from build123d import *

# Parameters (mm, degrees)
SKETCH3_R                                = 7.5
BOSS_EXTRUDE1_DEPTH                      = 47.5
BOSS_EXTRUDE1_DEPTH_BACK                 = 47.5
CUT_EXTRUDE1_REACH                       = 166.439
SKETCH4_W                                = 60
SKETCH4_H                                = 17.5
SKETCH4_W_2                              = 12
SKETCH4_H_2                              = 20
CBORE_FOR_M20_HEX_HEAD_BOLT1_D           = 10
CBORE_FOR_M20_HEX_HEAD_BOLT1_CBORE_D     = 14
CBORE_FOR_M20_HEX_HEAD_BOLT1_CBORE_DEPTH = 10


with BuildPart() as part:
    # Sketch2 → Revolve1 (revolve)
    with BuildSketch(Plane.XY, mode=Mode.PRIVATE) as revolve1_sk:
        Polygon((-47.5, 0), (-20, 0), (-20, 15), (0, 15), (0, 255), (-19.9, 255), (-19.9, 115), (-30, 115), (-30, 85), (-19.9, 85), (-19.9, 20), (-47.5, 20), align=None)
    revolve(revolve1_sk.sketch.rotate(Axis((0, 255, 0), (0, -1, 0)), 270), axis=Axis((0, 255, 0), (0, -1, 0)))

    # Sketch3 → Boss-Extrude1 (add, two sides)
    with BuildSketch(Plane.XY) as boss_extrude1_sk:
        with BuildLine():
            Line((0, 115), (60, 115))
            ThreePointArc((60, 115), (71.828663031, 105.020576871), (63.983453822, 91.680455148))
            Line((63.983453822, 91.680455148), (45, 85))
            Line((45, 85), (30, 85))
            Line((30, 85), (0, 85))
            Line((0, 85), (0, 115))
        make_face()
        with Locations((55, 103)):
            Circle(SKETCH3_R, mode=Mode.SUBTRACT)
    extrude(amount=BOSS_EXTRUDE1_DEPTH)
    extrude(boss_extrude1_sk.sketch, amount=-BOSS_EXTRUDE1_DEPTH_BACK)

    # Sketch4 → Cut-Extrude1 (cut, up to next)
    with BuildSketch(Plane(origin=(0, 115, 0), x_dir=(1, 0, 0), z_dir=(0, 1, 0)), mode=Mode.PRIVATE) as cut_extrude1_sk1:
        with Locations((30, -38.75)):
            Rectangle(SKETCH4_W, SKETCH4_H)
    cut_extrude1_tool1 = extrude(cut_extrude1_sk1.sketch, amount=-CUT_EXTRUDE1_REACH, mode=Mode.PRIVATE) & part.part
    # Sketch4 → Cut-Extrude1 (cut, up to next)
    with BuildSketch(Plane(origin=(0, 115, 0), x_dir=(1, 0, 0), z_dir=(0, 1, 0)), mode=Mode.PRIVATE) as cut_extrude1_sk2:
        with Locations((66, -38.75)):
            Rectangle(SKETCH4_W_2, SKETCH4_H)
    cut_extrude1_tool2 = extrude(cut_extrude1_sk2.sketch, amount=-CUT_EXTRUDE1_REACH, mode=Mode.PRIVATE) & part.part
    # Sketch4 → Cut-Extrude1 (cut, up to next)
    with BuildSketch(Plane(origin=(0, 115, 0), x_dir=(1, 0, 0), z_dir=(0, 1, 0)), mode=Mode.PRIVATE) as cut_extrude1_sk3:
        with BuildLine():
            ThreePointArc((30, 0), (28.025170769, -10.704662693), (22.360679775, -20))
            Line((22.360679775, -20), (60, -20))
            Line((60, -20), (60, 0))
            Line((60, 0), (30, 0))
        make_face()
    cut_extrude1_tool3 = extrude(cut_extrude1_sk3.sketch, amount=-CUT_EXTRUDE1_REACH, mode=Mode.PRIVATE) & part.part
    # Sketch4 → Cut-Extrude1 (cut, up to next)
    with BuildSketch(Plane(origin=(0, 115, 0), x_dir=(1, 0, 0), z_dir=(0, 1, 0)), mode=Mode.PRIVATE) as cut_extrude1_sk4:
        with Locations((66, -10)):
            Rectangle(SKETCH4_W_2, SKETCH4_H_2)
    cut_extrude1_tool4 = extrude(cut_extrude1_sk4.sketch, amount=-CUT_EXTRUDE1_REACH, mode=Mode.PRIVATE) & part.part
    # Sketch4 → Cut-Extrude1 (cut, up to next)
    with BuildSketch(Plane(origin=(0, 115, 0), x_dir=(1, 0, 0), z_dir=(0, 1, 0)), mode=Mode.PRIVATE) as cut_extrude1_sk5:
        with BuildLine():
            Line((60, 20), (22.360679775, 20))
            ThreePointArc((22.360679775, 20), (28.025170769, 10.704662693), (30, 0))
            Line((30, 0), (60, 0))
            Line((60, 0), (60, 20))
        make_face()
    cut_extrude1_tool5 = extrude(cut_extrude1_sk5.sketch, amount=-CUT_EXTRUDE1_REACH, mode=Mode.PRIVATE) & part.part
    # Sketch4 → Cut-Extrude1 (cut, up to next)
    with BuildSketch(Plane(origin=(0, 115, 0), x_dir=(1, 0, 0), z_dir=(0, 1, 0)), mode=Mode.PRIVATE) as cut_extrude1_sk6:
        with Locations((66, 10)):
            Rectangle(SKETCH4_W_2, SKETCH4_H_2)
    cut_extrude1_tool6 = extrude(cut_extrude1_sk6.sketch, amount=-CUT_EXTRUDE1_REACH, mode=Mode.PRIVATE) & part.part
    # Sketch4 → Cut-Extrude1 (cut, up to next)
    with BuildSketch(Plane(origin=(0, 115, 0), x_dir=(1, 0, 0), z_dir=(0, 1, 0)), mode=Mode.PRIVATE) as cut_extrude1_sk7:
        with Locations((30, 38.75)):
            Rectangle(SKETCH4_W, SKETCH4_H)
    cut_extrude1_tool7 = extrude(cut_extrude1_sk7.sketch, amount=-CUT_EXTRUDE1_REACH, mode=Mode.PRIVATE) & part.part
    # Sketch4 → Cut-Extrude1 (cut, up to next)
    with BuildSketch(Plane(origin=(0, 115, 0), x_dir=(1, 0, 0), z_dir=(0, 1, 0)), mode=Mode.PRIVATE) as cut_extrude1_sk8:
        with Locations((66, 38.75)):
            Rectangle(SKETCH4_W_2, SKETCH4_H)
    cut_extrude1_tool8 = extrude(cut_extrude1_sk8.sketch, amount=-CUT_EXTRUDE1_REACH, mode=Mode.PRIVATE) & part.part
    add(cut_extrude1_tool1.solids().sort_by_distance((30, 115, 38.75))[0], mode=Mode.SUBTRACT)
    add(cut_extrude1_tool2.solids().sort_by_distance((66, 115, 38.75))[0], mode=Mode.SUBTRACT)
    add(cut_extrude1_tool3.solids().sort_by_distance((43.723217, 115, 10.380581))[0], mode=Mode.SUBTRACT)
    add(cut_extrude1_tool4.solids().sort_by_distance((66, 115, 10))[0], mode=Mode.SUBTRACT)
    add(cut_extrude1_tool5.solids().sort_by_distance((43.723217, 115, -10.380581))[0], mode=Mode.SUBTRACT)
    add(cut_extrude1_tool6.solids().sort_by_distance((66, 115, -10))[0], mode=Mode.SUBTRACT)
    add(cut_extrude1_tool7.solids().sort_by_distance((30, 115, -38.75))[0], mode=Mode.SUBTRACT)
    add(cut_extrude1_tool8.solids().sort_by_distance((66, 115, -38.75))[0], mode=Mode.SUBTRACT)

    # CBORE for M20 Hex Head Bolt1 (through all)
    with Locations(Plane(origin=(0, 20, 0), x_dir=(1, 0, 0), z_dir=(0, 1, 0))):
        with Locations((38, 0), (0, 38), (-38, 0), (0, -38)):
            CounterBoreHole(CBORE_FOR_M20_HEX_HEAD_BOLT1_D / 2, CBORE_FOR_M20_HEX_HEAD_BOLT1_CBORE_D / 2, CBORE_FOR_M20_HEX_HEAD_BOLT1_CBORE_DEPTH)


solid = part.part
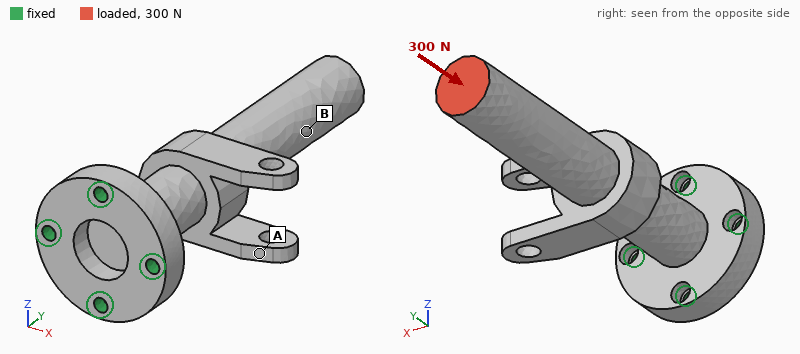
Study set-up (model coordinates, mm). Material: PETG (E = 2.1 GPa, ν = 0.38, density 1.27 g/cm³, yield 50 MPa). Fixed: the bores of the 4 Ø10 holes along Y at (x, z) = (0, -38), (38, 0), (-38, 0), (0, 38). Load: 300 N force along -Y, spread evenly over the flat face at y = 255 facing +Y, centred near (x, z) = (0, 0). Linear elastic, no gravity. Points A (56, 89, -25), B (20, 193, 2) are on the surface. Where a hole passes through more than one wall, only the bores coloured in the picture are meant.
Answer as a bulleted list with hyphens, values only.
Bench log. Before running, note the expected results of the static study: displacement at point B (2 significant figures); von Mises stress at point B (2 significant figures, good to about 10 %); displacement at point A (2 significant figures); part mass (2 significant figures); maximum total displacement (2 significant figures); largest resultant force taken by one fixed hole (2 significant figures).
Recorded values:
- 27 µm
- 0.24 MPa
- 17 µm
- 610 g
- 34 µm
- 94 N
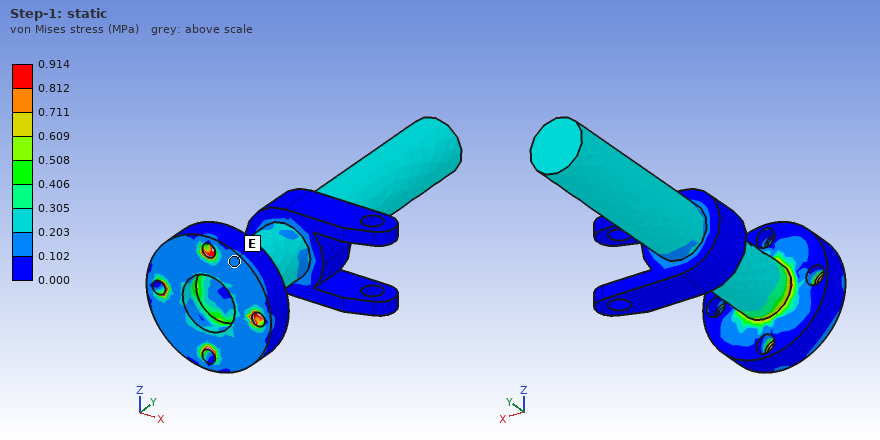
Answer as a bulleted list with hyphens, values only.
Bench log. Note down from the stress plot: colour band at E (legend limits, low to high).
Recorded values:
- 0.102 to 0.203 MPa
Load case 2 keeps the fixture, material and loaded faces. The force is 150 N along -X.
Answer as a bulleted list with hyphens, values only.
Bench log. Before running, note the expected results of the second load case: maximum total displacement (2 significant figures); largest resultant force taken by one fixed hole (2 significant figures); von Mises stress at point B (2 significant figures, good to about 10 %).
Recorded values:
- 3.2 mm
- 590 N
- 1.5 MPa
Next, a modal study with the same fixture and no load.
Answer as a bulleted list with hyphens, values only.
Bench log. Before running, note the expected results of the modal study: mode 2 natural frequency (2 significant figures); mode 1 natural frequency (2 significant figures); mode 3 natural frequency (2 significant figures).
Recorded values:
- 110 Hz
- 110 Hz
- 500 Hz
